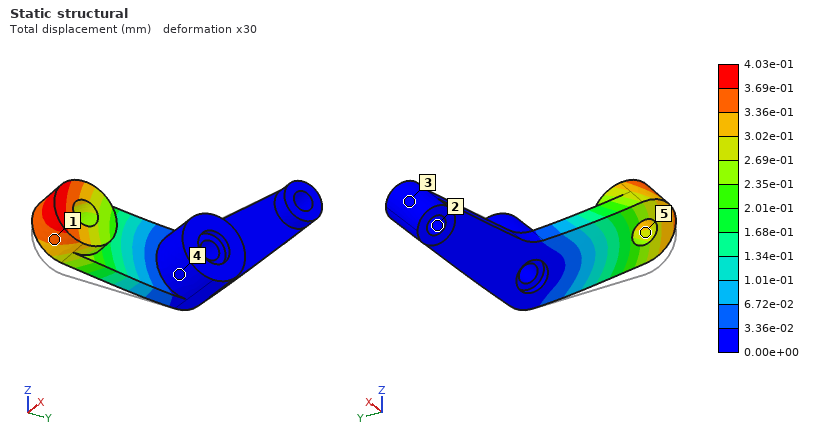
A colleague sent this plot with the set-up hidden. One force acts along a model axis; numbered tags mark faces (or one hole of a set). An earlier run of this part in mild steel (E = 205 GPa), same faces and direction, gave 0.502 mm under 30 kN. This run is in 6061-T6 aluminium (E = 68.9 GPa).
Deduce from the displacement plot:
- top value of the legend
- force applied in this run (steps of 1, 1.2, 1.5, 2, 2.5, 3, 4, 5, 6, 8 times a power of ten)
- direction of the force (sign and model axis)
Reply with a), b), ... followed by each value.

a) 4.03e-01 mm
b) 8 kN
c) +Z
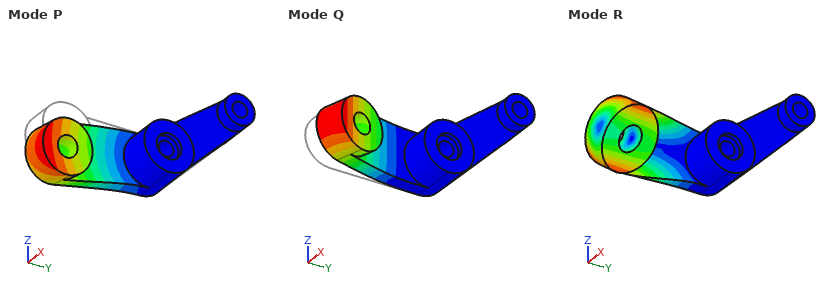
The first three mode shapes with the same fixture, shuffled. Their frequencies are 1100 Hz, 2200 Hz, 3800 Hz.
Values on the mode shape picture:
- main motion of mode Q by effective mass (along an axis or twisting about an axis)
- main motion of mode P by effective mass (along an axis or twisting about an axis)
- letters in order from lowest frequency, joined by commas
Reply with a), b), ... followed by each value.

a) along X
b) along Z
c) Q, P, R
